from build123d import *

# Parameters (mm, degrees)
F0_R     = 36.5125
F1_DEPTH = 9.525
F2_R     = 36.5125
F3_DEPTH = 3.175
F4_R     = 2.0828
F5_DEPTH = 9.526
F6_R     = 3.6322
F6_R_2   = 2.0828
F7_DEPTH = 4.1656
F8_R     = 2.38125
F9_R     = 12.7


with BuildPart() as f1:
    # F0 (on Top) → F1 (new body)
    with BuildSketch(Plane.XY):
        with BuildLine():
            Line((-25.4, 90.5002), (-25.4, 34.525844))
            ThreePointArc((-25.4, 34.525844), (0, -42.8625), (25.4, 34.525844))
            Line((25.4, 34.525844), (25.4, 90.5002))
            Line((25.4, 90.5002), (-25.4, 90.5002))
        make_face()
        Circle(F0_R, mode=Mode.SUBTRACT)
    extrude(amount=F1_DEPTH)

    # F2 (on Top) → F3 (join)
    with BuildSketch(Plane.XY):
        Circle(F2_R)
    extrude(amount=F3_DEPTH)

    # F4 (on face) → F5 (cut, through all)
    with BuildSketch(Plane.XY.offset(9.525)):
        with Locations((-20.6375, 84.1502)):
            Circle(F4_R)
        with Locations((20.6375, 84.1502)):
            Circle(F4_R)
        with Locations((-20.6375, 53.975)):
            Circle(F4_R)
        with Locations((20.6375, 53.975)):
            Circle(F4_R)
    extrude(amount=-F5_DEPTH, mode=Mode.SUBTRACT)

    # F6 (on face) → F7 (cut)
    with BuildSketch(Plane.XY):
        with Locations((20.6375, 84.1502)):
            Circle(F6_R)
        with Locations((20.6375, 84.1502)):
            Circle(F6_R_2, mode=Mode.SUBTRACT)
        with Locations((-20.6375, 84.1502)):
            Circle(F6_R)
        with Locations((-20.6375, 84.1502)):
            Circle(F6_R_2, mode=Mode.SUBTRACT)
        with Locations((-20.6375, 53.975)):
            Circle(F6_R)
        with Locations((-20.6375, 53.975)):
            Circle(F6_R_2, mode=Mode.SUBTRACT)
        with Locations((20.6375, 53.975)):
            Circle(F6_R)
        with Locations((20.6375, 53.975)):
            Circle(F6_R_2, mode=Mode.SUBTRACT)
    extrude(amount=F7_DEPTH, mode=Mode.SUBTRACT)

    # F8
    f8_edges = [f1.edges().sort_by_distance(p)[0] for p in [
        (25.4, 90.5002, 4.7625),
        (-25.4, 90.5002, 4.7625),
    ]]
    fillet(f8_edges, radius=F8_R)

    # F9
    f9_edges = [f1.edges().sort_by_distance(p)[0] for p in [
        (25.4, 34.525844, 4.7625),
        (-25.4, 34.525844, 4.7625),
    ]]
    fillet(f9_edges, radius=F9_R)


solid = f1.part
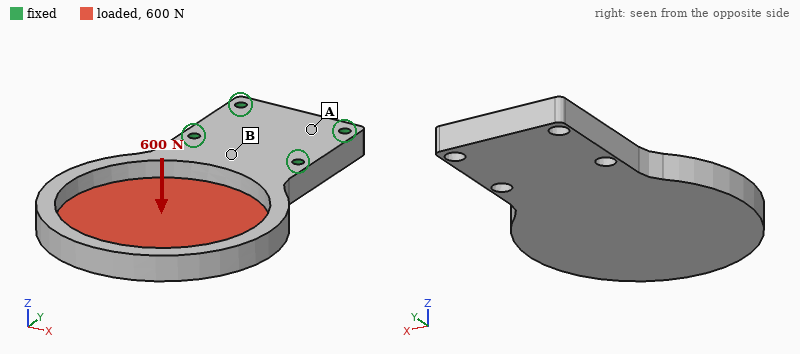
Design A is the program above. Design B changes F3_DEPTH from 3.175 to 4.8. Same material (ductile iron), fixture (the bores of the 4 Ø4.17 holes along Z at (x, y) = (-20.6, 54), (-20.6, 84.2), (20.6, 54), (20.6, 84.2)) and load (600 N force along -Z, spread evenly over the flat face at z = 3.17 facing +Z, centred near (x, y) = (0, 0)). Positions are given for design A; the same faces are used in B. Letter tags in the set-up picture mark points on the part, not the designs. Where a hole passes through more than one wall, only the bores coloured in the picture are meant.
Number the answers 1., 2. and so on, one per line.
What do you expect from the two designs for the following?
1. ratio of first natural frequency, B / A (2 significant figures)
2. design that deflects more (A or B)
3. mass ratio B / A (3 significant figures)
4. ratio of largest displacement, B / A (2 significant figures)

1. 1.0
2. A
3. 1.13
4. 0.82
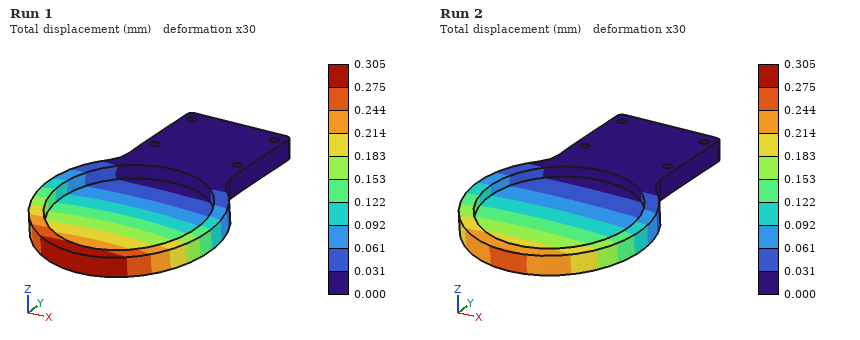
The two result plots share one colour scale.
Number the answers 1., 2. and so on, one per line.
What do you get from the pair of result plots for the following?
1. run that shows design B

1. Run 2
